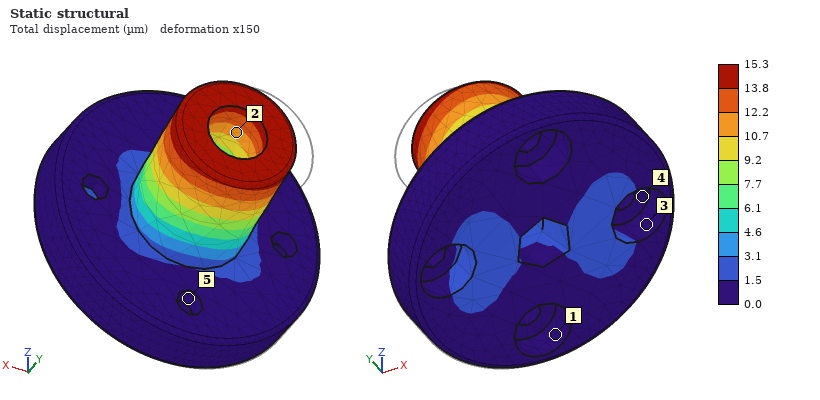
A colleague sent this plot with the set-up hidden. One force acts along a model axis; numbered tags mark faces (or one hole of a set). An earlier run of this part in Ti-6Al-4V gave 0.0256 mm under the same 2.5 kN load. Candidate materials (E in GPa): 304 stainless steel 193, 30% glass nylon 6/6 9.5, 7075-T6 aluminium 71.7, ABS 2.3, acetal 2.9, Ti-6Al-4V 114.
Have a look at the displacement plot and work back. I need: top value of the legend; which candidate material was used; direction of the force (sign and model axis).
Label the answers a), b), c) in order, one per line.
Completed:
a) 15.3 µm
b) 304 stainless steel
c) +X
